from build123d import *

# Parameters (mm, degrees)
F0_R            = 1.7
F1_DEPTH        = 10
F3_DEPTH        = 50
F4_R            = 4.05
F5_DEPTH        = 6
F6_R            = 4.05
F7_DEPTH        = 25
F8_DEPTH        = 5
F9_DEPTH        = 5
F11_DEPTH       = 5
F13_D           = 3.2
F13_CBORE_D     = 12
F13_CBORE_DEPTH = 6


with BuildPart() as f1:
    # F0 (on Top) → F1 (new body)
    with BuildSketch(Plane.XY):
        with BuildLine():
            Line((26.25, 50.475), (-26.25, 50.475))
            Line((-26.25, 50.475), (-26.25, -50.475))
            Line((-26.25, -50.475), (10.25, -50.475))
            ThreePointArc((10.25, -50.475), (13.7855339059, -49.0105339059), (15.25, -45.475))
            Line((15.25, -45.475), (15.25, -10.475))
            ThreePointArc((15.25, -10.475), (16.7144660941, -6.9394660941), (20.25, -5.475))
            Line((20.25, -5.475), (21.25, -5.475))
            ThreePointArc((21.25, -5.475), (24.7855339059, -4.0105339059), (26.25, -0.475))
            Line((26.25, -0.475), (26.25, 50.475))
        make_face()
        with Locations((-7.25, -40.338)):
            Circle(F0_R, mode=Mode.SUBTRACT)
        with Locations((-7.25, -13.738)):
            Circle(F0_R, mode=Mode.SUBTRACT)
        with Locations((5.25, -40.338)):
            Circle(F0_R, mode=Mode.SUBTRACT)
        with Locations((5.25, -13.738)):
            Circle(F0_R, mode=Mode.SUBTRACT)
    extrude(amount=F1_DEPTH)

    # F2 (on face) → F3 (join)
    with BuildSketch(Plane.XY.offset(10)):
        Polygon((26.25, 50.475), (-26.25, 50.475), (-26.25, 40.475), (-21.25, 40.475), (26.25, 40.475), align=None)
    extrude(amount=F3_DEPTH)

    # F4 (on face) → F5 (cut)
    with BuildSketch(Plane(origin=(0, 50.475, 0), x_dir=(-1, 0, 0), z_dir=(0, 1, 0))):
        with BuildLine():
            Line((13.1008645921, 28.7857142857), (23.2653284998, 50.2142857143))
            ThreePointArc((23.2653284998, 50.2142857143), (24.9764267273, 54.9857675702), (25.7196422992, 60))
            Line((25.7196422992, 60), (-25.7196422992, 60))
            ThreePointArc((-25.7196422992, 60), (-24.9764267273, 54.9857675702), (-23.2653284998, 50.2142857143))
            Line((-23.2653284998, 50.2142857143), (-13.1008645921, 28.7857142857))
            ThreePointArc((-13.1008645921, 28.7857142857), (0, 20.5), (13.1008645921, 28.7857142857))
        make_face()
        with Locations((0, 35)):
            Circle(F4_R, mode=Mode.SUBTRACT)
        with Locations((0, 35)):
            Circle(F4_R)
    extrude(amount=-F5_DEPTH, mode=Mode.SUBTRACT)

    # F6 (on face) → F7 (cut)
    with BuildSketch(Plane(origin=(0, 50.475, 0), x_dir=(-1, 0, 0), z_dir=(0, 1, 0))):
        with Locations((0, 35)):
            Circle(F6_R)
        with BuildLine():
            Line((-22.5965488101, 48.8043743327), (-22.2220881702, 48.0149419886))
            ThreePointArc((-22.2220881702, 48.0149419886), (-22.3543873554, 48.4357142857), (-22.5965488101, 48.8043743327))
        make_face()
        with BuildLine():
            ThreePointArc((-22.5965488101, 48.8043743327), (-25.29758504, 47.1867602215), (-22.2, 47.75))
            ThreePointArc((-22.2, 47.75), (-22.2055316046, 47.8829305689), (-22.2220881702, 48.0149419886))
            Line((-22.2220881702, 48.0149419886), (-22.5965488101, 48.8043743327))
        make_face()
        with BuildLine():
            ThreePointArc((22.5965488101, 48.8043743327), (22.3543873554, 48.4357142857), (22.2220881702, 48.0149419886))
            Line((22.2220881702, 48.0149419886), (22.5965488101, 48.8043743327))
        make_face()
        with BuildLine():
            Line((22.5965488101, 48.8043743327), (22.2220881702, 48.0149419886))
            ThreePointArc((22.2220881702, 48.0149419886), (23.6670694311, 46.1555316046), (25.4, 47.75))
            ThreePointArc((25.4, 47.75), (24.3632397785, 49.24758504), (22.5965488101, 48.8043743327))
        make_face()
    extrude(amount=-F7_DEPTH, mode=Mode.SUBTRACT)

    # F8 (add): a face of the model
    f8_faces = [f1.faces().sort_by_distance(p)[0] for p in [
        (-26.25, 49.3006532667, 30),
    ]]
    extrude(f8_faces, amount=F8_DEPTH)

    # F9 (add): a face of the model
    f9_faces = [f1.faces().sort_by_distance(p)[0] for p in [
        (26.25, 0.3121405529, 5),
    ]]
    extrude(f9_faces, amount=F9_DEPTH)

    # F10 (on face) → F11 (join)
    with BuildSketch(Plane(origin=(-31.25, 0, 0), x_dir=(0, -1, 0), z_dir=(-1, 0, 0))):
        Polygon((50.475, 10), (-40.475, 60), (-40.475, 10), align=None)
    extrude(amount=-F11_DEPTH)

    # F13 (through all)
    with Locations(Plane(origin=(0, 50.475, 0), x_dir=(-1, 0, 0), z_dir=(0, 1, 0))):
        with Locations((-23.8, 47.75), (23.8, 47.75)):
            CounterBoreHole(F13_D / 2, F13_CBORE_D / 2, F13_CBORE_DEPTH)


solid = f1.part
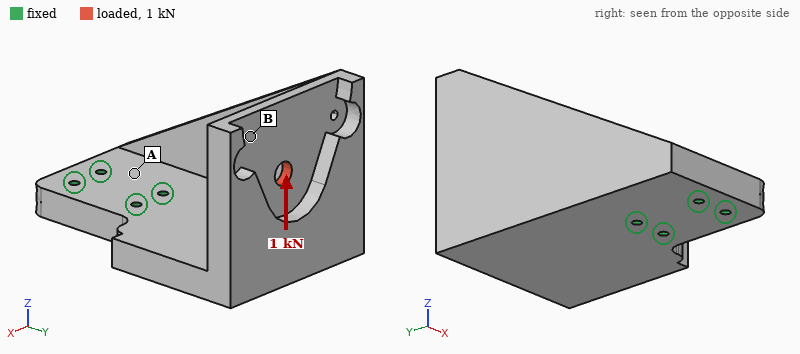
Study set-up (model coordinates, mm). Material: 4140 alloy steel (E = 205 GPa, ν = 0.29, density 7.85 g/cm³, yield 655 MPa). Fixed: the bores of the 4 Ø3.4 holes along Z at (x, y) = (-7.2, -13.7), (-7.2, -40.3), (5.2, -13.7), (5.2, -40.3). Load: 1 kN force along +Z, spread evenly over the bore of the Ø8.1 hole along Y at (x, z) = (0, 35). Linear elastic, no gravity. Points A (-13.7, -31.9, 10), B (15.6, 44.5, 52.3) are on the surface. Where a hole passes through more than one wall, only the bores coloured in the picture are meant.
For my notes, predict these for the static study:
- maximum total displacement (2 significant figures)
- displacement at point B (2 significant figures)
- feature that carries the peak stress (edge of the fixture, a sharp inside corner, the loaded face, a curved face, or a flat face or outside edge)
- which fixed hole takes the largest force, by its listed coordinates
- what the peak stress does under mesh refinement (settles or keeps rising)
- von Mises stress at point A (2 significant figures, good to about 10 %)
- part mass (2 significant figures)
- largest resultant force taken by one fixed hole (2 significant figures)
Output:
71 µm
60 µm
edge of the fixture
(-7.2, -13.7)
keeps rising
16 MPa
690 g
1.6 kN
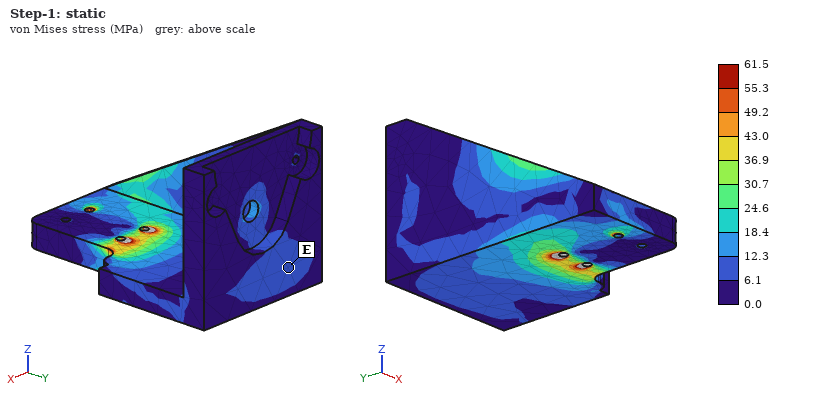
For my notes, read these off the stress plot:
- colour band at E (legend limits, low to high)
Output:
6.1 to 12.3 MPa
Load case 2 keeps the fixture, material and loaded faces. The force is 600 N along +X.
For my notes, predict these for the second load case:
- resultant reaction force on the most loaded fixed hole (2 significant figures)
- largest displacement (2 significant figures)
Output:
1.3 kN
41 µm
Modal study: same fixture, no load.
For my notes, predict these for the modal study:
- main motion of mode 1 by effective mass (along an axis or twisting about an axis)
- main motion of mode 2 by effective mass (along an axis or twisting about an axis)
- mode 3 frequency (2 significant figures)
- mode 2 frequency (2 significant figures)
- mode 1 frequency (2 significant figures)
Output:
along Z
along X
3100 Hz
1500 Hz
1200 Hz
